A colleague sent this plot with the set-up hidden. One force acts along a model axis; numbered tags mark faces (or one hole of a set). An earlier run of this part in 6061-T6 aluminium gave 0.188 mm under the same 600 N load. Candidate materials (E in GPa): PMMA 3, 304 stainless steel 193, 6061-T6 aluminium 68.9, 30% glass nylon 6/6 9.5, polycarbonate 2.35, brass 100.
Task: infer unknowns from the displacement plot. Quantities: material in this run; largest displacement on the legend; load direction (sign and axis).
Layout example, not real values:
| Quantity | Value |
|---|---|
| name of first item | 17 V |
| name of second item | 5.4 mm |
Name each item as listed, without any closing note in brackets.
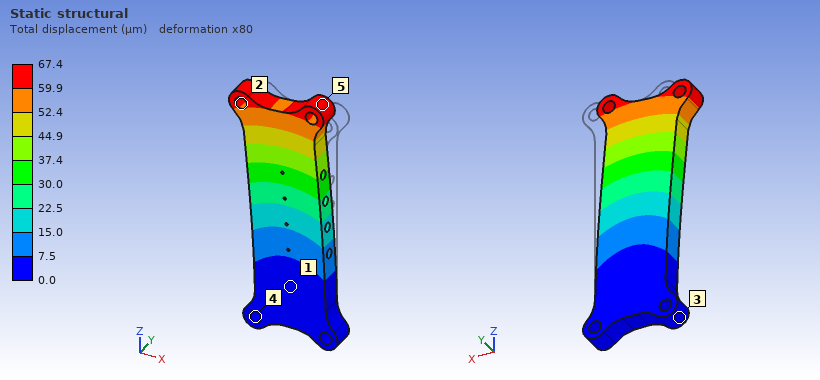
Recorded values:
| Quantity | Value |
|---|---|
| material in this run | 304 stainless steel |
| largest displacement on the legend | 67.4 µm |
| load direction | -X |
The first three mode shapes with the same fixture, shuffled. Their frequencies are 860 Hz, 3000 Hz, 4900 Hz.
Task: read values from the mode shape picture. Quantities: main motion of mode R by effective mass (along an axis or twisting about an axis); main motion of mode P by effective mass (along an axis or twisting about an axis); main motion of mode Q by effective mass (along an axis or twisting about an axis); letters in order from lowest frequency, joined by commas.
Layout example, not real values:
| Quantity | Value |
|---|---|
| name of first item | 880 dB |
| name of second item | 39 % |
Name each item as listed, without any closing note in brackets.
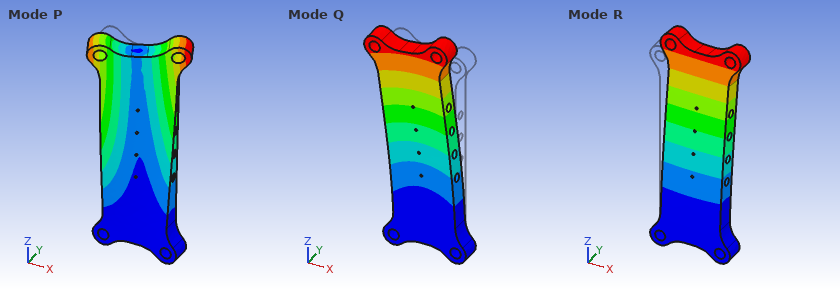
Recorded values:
| Quantity | Value |
|---|---|
| main motion of mode R by effective mass | along Y |
| main motion of mode P by effective mass | twisting about Z |
| main motion of mode Q by effective mass | along X |
| letters in order from lowest frequency, joined by commas | R, Q, P |
